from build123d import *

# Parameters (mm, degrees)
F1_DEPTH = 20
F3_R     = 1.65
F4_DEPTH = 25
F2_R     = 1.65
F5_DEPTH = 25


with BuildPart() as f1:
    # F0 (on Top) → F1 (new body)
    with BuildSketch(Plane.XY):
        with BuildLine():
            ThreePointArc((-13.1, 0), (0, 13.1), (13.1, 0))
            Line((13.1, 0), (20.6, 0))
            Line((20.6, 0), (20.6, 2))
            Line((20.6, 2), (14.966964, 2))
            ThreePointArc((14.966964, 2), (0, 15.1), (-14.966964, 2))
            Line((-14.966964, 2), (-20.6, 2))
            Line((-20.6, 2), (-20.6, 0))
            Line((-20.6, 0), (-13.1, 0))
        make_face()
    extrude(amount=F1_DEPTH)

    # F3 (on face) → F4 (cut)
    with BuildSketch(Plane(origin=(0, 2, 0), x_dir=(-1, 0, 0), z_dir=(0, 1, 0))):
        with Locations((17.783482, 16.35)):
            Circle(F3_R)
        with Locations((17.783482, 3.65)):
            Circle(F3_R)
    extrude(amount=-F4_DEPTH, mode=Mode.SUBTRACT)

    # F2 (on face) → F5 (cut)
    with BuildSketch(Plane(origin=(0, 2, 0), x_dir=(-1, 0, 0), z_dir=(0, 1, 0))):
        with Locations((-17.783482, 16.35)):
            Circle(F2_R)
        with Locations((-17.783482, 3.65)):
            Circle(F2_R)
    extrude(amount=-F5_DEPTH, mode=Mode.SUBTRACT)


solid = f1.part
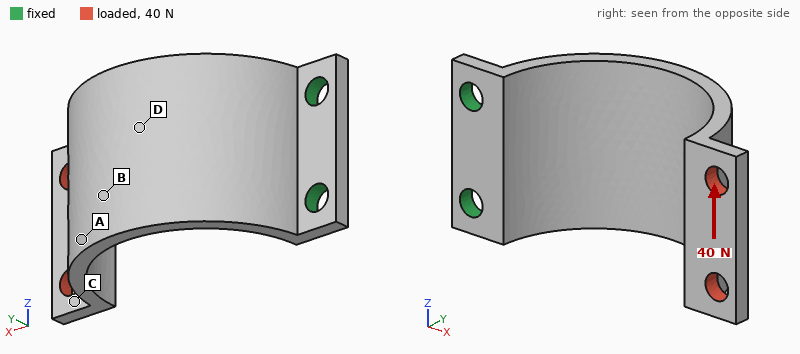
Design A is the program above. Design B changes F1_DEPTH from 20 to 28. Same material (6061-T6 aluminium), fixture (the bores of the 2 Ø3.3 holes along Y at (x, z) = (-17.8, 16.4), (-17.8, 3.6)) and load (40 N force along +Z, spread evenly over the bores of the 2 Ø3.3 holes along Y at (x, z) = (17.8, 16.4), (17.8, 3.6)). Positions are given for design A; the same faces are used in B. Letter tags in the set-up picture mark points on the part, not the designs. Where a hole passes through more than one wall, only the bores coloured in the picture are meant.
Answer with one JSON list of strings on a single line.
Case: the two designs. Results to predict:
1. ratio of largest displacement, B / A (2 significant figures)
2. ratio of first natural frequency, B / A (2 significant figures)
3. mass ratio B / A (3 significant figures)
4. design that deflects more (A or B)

["0.71", "0.97", "1.41", "A"]
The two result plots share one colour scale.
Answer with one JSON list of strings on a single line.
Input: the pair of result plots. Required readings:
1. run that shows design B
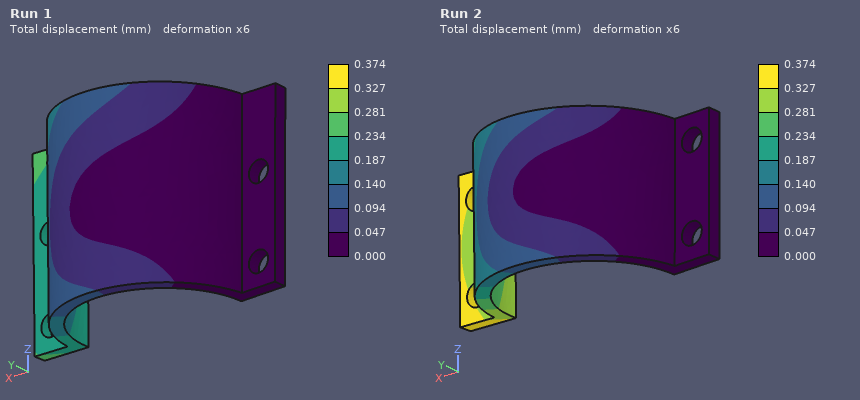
["Run 1"]
